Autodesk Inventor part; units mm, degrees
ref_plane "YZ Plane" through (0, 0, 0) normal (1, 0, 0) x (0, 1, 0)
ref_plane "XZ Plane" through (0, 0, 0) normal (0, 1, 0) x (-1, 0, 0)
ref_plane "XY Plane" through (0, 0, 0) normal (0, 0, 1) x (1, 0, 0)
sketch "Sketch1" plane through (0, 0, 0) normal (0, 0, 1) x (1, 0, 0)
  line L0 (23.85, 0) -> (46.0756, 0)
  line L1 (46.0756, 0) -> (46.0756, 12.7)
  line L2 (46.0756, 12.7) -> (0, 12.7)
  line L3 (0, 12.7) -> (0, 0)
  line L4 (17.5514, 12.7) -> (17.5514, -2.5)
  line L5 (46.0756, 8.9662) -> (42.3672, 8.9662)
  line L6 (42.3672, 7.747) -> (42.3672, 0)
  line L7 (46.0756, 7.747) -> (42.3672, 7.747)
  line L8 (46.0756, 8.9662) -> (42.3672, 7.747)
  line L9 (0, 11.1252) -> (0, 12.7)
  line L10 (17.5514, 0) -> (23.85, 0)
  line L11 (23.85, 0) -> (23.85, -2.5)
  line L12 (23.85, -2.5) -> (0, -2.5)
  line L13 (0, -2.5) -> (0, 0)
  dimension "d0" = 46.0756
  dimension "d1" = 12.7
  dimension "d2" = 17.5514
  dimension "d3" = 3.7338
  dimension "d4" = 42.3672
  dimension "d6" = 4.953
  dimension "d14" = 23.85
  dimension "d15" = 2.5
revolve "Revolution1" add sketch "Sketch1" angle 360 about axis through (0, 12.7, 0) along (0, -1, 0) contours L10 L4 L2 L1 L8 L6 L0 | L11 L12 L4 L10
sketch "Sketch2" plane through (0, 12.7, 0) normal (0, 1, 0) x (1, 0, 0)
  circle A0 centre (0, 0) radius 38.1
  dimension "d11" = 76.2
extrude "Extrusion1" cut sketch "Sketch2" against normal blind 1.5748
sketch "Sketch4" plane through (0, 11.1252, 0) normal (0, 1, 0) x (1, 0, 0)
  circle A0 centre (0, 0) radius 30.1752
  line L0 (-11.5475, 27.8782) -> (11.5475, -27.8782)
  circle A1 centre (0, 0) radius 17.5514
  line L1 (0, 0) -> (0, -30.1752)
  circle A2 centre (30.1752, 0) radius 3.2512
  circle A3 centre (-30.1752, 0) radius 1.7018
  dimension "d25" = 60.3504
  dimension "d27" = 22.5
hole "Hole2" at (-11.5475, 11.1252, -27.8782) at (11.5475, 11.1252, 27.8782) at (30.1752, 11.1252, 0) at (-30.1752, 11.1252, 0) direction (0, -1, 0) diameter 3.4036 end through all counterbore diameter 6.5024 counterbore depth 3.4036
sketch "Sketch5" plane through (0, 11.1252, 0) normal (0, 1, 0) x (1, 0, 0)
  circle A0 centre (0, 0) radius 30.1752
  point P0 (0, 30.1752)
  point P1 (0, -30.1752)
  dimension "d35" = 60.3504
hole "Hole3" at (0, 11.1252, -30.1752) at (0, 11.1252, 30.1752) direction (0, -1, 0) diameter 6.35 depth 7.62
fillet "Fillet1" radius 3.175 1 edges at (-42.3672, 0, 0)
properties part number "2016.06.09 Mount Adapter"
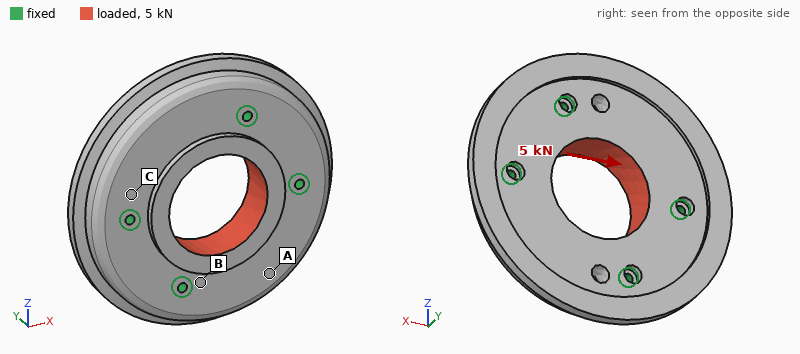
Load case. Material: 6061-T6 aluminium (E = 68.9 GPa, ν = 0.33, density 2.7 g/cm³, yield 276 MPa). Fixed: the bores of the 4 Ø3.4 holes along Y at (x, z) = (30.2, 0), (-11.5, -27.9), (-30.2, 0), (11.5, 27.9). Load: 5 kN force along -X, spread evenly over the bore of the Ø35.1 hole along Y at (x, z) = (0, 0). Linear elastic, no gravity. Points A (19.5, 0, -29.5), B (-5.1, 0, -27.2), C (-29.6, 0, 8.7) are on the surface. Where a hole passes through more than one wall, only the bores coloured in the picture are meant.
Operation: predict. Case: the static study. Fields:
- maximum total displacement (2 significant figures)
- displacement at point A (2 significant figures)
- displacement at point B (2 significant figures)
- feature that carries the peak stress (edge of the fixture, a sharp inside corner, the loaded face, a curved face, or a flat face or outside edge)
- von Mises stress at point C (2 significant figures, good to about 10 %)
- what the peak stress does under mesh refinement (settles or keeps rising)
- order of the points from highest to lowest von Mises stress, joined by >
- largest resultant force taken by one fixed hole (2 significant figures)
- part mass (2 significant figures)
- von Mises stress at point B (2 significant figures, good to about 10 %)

2.7 µm
1.8 µm
0.71 µm
edge of the fixture
3.8 MPa
keeps rising
B > C > A
1.3 kN
160 g
7.9 MPa
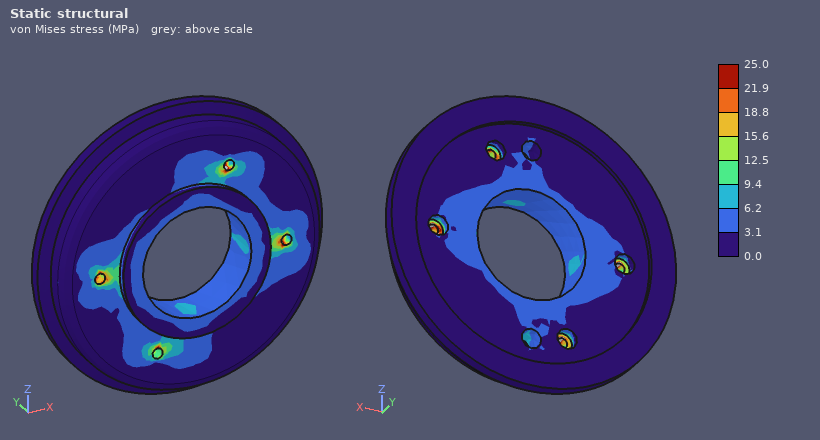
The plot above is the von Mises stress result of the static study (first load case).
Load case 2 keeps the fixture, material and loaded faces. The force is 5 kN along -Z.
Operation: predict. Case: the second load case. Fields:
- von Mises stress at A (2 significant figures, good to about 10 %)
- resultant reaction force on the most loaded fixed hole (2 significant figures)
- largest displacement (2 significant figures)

2.6 MPa
1.3 kN
3.4 µm
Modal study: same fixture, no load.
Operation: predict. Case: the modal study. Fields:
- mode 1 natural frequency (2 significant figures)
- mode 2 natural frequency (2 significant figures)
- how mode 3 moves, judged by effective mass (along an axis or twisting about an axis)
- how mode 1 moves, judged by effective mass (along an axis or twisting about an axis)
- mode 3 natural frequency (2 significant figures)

7300 Hz
8000 Hz
along Y
along Y
15 kHz
